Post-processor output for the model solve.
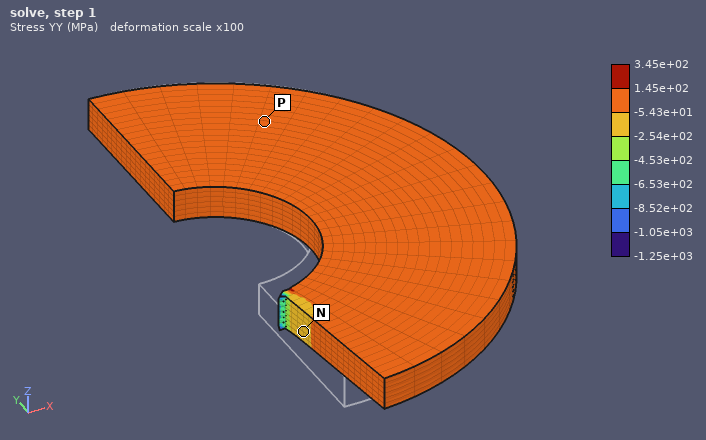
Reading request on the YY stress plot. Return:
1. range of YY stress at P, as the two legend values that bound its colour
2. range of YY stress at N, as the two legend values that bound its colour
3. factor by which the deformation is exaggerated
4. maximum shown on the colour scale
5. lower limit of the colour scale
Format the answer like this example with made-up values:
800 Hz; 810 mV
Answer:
-5.43e+01 to 1.45e+02 MPa; -2.54e+02 to -5.43e+01 MPa; 100; 3.45e+02 MPa; -1.25e+03 MPa
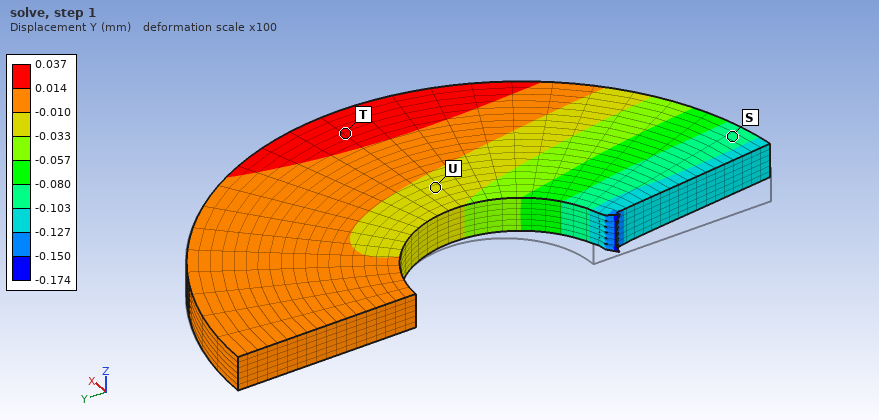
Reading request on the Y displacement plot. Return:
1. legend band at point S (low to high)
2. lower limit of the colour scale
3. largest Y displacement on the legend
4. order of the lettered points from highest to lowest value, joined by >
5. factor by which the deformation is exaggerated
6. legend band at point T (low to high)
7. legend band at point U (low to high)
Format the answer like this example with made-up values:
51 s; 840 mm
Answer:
-0.103 to -0.080 mm; -0.174 mm; 0.037 mm; T > U > S; 100; 0.014 to 0.037 mm; -0.033 to -0.010 mm
